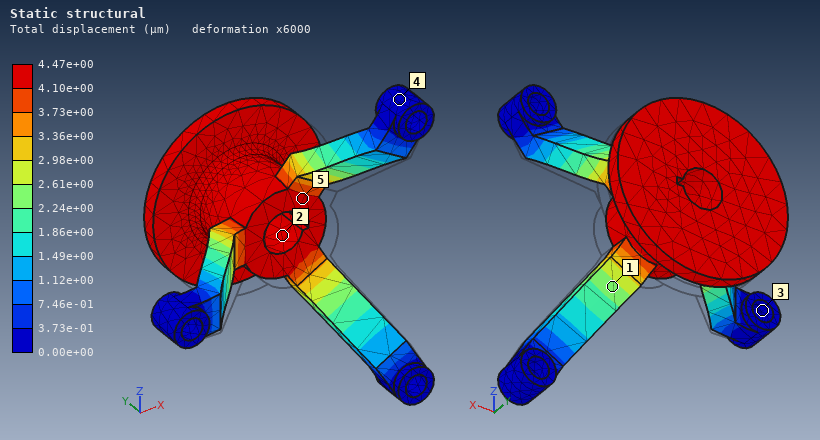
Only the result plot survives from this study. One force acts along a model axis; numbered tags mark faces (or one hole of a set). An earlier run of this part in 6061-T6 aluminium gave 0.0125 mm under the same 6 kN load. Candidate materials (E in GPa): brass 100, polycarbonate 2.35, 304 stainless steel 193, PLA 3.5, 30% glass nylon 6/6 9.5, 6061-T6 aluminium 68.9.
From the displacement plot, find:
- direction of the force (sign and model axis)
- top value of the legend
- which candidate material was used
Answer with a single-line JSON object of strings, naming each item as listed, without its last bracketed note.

{"direction of the force": "+Y", "top value of the legend": "4.47e+00 µm", "which candidate material was used": "304 stainless steel"}
